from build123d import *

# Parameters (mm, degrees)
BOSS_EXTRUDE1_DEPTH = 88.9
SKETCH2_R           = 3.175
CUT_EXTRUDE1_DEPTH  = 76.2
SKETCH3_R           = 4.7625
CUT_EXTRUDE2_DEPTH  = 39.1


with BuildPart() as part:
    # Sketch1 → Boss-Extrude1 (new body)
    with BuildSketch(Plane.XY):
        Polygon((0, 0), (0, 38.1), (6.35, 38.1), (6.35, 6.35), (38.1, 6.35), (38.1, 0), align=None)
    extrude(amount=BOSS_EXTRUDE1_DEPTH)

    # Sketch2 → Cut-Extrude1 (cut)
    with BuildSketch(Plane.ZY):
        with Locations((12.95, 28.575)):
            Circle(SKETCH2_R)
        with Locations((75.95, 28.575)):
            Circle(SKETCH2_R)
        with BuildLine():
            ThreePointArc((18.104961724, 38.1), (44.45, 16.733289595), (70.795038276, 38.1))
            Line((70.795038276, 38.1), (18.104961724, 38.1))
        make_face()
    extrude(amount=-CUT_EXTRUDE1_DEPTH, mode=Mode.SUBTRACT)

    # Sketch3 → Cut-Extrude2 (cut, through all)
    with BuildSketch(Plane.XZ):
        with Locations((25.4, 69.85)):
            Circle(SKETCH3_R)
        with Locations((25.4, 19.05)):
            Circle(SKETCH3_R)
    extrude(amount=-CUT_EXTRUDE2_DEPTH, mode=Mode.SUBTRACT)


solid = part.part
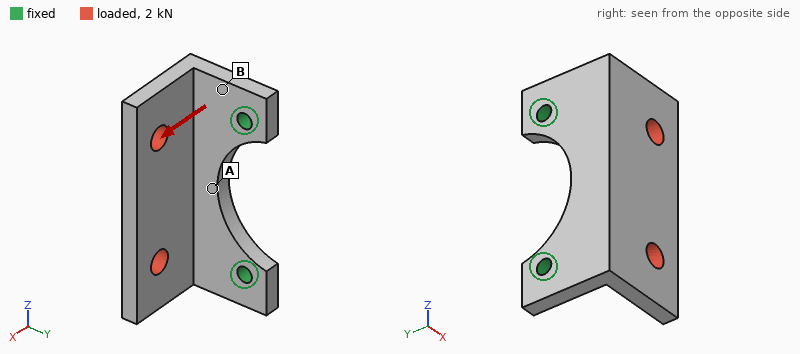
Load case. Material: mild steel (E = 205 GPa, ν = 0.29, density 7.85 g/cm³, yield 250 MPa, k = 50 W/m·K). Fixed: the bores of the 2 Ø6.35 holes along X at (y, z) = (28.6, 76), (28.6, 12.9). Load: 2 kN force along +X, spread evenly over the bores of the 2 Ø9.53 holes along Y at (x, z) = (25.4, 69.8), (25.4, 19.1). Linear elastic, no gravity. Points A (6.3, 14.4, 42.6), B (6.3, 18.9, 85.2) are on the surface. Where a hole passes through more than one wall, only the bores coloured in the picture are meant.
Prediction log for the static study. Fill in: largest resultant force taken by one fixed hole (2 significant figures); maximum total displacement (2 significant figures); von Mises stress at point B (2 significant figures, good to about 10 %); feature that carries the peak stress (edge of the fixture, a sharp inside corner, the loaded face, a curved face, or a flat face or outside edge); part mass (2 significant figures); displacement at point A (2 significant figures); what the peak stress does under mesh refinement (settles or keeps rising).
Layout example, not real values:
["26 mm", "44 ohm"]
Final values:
["1.0 kN", "0.11 mm", "78 MPa", "edge of the fixture", "260 g", "0.021 mm", "keeps rising"]
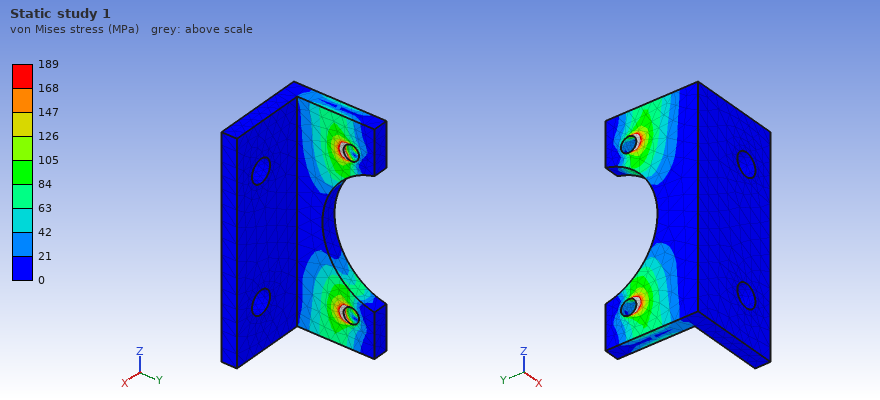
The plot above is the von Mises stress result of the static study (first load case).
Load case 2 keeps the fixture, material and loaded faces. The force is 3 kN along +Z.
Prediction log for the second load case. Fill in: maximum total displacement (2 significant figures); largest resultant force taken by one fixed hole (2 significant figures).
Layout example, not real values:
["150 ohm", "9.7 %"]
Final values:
["52 µm", "2.0 kN"]
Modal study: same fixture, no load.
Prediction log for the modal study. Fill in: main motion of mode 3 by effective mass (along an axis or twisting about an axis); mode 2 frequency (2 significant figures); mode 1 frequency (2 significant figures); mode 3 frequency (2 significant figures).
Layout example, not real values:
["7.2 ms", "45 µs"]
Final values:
["along X", "3100 Hz", "1600 Hz", "4700 Hz"]
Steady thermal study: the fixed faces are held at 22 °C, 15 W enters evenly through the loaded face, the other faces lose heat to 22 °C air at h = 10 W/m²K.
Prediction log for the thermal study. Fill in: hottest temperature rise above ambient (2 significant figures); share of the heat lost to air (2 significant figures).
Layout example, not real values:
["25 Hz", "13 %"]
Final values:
["32 K", "15 %"]
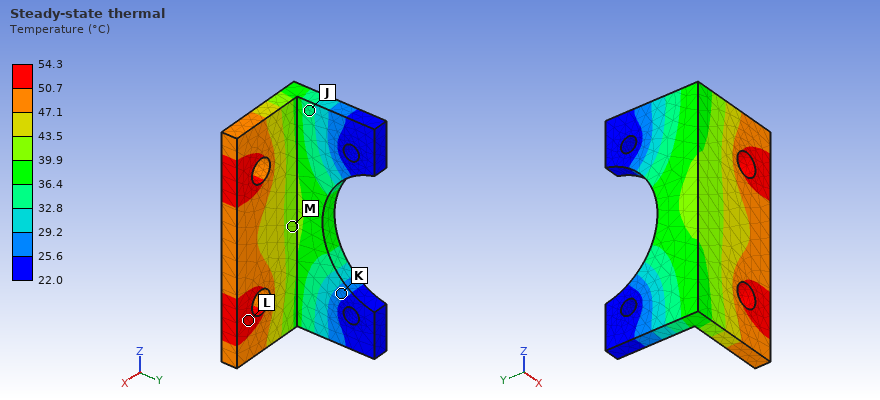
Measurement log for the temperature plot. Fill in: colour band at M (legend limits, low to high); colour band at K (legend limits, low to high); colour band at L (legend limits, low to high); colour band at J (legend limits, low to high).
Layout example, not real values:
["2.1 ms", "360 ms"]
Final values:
["39.9 to 43.5 °C", "25.6 to 29.2 °C", "50.7 to 54.3 °C", "32.8 to 36.4 °C"]
